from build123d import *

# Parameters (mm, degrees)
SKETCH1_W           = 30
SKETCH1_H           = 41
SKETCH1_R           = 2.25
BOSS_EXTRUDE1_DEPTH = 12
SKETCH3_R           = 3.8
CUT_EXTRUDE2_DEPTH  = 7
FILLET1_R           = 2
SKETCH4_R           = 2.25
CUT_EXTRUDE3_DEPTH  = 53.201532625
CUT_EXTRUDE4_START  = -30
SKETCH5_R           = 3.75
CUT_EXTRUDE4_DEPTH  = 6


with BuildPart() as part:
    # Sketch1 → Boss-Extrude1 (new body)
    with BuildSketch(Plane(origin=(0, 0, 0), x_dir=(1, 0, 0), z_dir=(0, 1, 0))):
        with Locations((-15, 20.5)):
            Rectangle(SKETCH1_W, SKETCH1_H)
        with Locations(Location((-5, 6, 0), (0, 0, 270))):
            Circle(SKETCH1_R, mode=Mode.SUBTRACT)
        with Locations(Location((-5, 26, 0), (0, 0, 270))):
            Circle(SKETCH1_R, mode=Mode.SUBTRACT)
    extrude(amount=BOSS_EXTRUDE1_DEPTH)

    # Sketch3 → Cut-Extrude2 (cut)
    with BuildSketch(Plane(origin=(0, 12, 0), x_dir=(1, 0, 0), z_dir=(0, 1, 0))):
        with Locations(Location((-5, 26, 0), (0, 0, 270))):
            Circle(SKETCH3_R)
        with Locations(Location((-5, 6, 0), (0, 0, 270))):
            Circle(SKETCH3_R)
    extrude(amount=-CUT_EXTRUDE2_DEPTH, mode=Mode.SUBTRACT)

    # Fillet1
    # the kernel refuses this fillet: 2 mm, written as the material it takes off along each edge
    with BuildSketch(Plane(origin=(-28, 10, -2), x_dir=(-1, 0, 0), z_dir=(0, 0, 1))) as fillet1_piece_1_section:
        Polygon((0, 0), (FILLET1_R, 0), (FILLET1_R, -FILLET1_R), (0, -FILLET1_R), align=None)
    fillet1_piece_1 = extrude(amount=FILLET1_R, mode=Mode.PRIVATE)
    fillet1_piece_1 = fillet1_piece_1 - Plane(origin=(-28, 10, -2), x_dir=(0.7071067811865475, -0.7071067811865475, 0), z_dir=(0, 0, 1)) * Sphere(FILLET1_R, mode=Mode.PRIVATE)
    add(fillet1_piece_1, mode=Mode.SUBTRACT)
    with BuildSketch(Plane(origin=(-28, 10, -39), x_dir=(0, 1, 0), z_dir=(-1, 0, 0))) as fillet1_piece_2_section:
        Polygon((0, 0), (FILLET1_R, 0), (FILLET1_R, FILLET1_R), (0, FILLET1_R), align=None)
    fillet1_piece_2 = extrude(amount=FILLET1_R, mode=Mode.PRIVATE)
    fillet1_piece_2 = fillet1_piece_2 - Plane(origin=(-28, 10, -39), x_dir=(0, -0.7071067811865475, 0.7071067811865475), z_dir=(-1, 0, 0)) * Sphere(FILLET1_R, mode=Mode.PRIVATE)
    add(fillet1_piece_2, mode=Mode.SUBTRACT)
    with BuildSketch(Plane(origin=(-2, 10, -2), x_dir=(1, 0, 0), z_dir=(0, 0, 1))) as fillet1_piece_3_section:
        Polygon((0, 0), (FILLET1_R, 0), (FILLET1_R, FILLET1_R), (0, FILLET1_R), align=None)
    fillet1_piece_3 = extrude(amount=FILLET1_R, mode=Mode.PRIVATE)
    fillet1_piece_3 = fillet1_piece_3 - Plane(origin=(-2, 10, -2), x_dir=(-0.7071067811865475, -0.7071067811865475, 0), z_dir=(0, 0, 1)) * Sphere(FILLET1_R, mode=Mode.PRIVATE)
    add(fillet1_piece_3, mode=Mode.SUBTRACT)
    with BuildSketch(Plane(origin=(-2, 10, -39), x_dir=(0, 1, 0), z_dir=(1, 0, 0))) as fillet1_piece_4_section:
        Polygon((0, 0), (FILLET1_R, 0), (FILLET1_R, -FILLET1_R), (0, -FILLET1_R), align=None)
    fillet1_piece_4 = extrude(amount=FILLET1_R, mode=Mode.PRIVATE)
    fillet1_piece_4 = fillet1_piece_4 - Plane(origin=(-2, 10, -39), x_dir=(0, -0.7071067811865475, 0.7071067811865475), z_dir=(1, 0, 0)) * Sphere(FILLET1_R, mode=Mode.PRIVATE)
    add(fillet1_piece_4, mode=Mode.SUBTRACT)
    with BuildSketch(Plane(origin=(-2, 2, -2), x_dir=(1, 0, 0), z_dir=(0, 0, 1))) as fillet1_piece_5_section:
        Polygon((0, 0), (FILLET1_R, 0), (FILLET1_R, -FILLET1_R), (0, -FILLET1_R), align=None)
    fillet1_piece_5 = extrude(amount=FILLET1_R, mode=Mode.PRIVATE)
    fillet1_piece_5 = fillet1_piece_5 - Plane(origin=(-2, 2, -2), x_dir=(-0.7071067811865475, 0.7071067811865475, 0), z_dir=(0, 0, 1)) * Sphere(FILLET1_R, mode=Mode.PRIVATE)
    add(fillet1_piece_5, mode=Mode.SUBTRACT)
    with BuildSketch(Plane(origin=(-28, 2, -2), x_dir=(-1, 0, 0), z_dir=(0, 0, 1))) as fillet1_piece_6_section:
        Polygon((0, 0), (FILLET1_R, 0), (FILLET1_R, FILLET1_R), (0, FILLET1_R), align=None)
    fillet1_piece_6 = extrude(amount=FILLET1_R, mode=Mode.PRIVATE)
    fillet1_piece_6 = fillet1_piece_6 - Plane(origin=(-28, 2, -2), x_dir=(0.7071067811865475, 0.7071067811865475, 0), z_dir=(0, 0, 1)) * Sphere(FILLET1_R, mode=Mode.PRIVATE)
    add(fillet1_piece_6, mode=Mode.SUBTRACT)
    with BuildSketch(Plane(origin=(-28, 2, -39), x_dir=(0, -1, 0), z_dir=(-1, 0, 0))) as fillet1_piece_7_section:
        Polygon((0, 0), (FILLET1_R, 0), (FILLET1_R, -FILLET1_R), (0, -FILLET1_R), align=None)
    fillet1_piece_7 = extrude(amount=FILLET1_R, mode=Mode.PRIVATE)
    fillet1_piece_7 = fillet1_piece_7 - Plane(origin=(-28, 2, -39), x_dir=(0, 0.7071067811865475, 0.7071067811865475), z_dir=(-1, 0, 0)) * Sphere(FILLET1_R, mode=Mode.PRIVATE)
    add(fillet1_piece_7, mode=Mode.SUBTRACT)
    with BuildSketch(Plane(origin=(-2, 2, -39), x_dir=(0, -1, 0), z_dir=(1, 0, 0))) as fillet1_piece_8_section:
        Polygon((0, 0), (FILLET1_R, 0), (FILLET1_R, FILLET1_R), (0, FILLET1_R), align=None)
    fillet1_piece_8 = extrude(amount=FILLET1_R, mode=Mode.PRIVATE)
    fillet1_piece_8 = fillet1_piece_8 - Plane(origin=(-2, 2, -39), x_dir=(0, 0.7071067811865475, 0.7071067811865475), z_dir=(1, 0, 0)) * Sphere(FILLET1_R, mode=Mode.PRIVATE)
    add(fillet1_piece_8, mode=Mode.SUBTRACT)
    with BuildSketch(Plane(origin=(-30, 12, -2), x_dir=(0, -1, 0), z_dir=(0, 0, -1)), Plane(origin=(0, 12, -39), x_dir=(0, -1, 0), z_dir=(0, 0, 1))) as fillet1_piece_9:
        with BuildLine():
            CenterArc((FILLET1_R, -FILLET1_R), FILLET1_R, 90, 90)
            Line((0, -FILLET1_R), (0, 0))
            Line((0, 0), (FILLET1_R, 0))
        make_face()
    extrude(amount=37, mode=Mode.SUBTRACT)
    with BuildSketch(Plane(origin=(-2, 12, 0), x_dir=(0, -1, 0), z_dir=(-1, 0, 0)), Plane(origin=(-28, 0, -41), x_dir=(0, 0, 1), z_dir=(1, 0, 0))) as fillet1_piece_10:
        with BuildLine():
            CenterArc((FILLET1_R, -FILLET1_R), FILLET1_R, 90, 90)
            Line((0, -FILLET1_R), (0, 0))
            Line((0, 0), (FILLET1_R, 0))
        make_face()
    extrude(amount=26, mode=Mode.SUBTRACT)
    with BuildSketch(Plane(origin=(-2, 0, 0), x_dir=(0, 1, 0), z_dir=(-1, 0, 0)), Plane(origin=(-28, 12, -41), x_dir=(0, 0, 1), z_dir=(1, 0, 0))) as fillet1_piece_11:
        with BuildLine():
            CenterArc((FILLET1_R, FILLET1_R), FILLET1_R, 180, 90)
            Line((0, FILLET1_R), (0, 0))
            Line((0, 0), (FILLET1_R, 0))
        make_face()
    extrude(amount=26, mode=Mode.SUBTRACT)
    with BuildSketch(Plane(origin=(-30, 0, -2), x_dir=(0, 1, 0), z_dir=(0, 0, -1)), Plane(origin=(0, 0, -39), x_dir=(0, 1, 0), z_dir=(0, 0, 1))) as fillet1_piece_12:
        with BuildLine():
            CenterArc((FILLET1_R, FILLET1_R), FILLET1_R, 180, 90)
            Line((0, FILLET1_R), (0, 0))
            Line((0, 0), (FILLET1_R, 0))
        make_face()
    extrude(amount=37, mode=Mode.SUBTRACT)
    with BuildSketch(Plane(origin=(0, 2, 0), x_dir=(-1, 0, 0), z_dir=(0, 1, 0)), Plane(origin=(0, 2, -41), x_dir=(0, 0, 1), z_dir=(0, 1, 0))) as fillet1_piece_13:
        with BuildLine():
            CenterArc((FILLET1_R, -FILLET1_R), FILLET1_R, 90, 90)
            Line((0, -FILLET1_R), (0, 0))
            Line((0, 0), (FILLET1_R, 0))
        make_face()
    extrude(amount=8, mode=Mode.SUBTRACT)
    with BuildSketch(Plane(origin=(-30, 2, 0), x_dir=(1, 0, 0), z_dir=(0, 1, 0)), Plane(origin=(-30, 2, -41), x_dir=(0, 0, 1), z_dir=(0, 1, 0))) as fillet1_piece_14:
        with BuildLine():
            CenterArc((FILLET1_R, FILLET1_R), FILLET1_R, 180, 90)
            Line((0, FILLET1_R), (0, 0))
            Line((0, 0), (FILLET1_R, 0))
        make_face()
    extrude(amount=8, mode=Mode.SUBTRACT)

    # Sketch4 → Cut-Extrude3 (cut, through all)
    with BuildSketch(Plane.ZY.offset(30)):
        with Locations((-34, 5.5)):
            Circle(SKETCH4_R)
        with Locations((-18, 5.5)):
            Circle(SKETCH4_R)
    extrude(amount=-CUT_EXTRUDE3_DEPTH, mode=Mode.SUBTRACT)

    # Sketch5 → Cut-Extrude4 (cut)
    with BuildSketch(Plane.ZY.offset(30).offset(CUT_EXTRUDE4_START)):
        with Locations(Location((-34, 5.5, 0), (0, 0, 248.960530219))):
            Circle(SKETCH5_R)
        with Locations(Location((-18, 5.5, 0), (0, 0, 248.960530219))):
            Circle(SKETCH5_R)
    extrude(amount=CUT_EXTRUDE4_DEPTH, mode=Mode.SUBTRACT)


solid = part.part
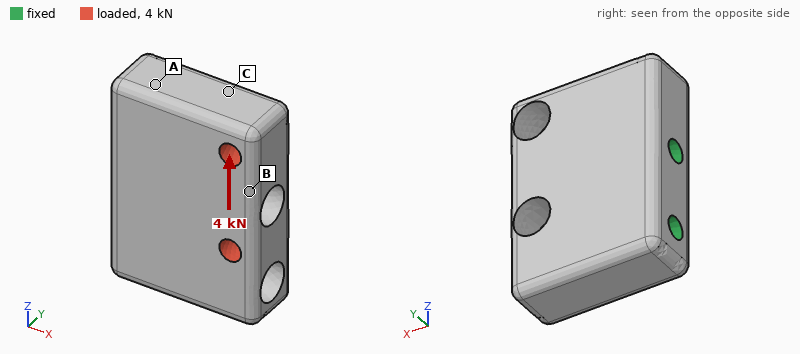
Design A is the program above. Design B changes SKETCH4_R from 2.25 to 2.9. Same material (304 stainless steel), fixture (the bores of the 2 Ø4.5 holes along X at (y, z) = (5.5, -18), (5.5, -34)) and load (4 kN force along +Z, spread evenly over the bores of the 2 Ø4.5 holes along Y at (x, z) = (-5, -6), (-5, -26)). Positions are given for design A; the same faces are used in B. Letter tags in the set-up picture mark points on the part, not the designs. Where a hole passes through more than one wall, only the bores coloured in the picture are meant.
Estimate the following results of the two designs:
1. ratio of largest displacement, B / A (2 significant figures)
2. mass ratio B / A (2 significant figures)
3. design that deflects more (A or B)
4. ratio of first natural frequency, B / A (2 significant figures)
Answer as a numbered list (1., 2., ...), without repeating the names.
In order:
1. 0.91
2. 0.96
3. A
4. 1.1
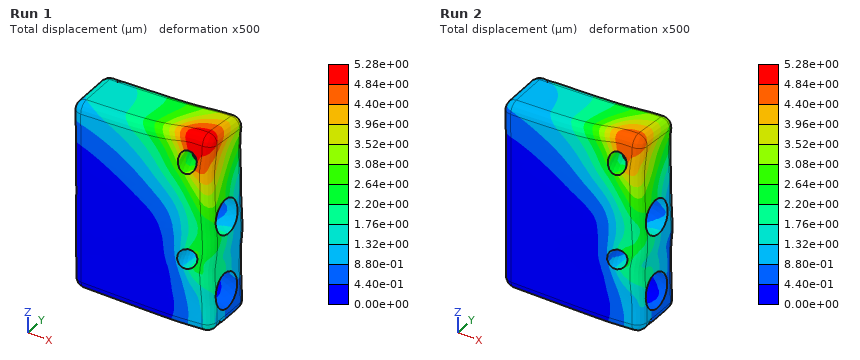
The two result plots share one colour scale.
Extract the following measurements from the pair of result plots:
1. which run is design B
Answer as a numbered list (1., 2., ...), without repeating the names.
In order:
1. Run 2
